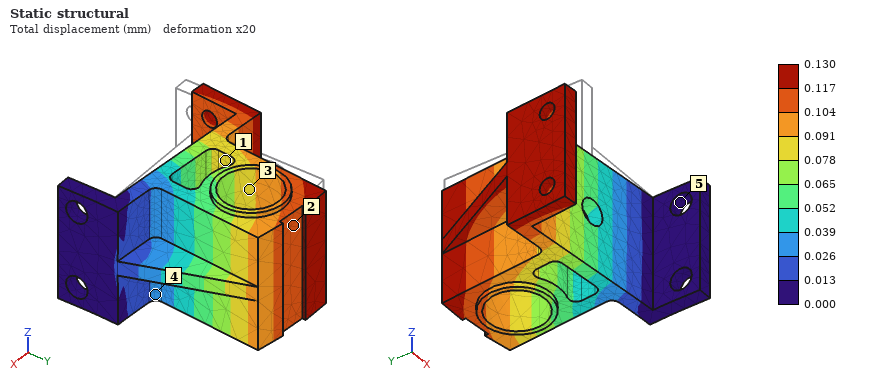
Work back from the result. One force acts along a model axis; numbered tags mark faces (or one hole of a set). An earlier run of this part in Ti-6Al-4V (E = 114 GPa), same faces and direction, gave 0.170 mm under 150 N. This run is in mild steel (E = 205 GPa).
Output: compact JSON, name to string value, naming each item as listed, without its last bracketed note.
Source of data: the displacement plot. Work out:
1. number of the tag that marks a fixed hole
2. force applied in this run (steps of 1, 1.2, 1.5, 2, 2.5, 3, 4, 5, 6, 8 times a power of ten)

{"number of the tag that marks a fixed hole": "5", "force applied in this run": "200 N"}
